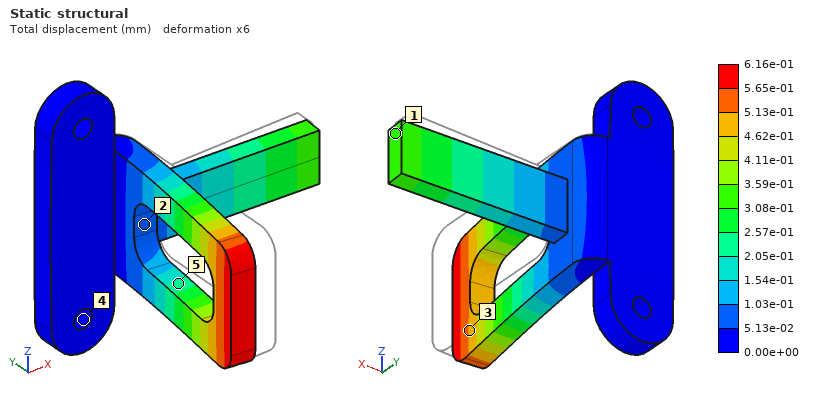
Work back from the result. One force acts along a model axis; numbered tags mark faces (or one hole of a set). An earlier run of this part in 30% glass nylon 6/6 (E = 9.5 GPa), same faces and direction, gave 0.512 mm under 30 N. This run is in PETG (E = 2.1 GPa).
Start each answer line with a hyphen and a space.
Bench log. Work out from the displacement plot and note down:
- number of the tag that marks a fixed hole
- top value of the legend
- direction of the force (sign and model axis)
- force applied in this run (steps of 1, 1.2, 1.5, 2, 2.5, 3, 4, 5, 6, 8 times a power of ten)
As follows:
- 4
- 6.16e-01 mm
- -X
- 8 N
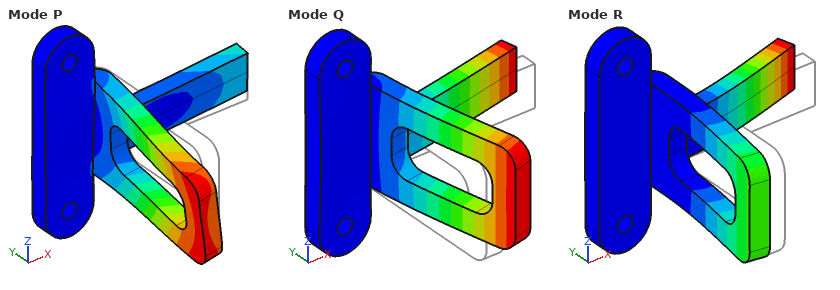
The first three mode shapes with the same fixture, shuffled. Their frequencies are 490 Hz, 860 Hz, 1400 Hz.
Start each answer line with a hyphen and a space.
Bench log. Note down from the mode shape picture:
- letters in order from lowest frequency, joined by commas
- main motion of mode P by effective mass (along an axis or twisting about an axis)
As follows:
- Q, R, P
- along Z
